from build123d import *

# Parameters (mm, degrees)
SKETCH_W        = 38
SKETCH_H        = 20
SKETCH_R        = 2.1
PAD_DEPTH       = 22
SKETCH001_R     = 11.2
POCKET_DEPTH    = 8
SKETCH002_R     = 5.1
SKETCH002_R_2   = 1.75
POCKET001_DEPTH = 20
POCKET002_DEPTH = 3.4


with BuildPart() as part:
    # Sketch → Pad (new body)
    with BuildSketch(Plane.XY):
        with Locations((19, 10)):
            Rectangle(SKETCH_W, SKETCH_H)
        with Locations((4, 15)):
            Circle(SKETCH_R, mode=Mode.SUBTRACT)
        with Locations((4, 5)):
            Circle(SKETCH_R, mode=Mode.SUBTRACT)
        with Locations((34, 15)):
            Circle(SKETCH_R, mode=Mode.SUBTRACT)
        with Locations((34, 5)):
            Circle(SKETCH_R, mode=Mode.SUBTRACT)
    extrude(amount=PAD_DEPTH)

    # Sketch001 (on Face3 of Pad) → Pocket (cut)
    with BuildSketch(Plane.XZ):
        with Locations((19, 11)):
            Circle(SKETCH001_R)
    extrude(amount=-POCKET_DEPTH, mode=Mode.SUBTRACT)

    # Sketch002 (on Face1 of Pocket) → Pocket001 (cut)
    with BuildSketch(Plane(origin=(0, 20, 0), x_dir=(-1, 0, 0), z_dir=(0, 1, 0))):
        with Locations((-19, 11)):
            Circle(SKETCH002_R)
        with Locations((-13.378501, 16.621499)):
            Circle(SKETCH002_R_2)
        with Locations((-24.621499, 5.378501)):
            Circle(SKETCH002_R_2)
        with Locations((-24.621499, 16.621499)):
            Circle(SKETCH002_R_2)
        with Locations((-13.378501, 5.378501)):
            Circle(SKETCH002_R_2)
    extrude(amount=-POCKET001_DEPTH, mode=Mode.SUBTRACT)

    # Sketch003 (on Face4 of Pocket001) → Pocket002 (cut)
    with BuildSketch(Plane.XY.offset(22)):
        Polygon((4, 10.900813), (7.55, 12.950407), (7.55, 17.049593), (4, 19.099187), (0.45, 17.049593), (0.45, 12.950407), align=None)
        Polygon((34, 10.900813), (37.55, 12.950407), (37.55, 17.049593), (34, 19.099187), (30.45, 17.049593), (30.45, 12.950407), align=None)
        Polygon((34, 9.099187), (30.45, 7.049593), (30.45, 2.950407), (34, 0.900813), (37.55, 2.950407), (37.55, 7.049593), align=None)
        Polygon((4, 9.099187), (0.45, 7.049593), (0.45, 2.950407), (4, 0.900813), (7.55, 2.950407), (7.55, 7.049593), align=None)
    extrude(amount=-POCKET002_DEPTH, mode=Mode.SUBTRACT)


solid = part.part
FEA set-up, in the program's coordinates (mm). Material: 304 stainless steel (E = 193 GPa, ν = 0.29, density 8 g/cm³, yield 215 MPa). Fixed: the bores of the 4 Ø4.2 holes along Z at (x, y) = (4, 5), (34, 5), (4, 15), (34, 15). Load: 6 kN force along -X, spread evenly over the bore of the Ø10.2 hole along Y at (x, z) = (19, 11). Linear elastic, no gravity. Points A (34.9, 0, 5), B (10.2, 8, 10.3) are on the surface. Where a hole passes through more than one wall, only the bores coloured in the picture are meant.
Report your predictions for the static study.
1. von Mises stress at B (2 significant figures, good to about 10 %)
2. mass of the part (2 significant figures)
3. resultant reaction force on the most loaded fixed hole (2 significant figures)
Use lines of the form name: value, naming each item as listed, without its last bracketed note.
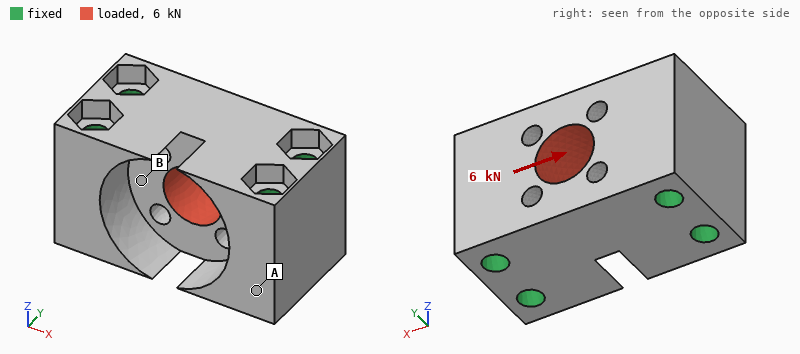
von Mises stress at B: 17 MPa
mass of the part: 84 g
resultant reaction force on the most loaded fixed hole: 2.4 kN
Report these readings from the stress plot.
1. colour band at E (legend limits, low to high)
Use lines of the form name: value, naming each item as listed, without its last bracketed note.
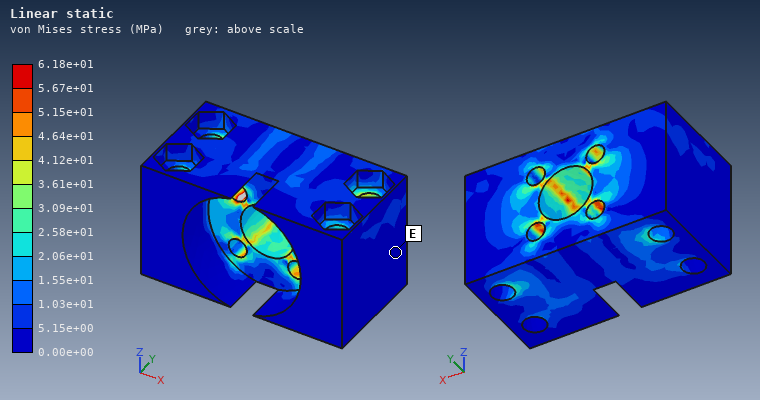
colour band at E: 0.00e+00 to 5.15e+00 MPa
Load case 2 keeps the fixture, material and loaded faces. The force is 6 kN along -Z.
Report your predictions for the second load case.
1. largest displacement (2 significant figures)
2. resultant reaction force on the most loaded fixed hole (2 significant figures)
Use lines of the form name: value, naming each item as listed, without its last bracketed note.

largest displacement: 3.5 µm
resultant reaction force on the most loaded fixed hole: 2.3 kN
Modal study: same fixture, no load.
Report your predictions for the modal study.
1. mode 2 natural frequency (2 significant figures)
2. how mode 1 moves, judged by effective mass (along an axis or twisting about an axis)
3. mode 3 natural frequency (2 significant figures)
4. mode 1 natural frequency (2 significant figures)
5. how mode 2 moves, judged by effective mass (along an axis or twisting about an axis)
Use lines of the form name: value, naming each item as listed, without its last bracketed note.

mode 2 natural frequency: 50 kHz
how mode 1 moves, judged by effective mass: along Y
mode 3 natural frequency: 54 kHz
mode 1 natural frequency: 46 kHz
how mode 2 moves, judged by effective mass: along Z
